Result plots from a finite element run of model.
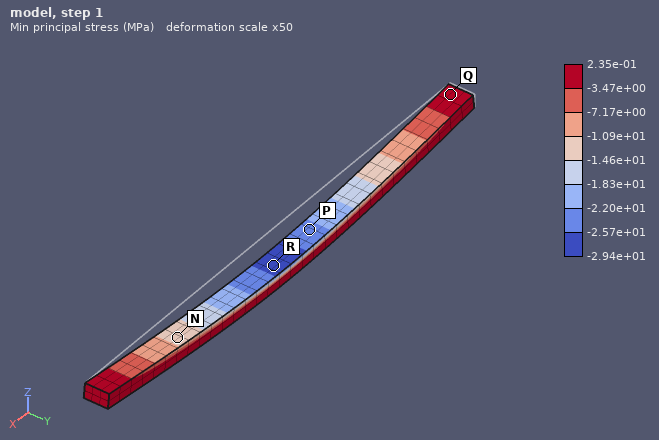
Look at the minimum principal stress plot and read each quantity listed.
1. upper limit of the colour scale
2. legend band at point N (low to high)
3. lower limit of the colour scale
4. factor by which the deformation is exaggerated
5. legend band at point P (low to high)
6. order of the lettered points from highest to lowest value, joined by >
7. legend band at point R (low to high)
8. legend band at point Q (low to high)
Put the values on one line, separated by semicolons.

2.35e-01 MPa; -1.46e+01 to -1.09e+01 MPa; -2.94e+01 MPa; 50; -2.57e+01 to -2.20e+01 MPa; Q > N > P > R; -2.94e+01 to -2.57e+01 MPa; -3.47e+00 to 2.35e-01 MPa
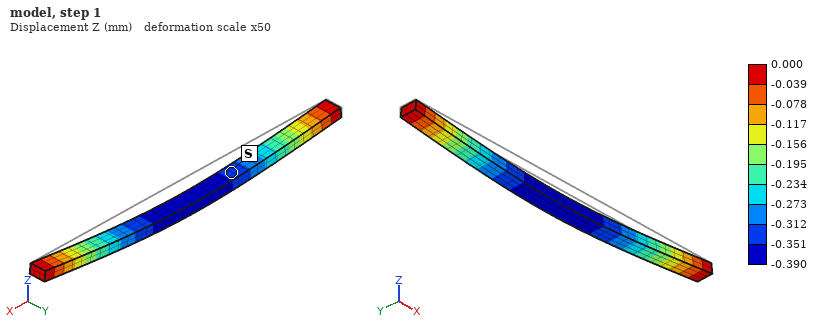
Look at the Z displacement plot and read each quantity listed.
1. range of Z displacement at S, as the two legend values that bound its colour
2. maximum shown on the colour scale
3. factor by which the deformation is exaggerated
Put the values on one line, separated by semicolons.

-0.351 to -0.312 mm; 0.000 mm; 50
